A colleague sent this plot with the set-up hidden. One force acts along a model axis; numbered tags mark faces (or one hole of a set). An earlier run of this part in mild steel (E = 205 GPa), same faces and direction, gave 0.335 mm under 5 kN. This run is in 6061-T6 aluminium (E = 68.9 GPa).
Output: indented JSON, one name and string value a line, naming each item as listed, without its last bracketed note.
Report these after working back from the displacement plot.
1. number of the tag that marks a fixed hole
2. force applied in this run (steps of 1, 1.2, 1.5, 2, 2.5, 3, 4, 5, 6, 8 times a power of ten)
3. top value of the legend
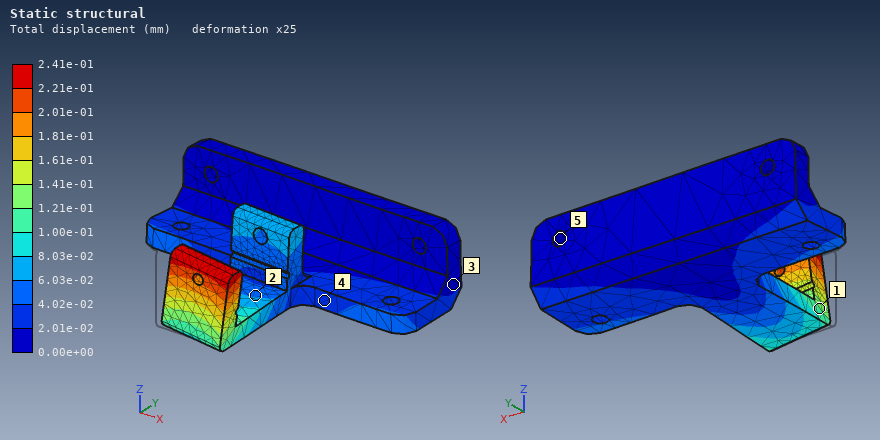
{
  "number of the tag that marks a fixed hole": "5",
  "force applied in this run": "1.2 kN",
  "top value of the legend": "2.41e-01 mm"
}
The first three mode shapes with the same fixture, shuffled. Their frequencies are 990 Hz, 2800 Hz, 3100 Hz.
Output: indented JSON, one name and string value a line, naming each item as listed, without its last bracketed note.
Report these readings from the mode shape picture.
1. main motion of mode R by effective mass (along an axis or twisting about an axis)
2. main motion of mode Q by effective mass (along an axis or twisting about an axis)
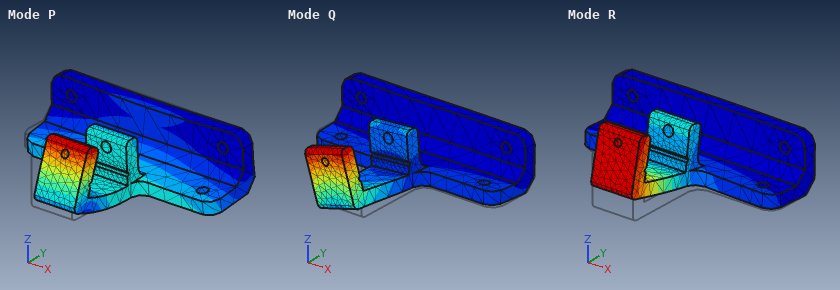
{
  "main motion of mode R by effective mass": "along Z",
  "main motion of mode Q by effective mass": "along X"
}
